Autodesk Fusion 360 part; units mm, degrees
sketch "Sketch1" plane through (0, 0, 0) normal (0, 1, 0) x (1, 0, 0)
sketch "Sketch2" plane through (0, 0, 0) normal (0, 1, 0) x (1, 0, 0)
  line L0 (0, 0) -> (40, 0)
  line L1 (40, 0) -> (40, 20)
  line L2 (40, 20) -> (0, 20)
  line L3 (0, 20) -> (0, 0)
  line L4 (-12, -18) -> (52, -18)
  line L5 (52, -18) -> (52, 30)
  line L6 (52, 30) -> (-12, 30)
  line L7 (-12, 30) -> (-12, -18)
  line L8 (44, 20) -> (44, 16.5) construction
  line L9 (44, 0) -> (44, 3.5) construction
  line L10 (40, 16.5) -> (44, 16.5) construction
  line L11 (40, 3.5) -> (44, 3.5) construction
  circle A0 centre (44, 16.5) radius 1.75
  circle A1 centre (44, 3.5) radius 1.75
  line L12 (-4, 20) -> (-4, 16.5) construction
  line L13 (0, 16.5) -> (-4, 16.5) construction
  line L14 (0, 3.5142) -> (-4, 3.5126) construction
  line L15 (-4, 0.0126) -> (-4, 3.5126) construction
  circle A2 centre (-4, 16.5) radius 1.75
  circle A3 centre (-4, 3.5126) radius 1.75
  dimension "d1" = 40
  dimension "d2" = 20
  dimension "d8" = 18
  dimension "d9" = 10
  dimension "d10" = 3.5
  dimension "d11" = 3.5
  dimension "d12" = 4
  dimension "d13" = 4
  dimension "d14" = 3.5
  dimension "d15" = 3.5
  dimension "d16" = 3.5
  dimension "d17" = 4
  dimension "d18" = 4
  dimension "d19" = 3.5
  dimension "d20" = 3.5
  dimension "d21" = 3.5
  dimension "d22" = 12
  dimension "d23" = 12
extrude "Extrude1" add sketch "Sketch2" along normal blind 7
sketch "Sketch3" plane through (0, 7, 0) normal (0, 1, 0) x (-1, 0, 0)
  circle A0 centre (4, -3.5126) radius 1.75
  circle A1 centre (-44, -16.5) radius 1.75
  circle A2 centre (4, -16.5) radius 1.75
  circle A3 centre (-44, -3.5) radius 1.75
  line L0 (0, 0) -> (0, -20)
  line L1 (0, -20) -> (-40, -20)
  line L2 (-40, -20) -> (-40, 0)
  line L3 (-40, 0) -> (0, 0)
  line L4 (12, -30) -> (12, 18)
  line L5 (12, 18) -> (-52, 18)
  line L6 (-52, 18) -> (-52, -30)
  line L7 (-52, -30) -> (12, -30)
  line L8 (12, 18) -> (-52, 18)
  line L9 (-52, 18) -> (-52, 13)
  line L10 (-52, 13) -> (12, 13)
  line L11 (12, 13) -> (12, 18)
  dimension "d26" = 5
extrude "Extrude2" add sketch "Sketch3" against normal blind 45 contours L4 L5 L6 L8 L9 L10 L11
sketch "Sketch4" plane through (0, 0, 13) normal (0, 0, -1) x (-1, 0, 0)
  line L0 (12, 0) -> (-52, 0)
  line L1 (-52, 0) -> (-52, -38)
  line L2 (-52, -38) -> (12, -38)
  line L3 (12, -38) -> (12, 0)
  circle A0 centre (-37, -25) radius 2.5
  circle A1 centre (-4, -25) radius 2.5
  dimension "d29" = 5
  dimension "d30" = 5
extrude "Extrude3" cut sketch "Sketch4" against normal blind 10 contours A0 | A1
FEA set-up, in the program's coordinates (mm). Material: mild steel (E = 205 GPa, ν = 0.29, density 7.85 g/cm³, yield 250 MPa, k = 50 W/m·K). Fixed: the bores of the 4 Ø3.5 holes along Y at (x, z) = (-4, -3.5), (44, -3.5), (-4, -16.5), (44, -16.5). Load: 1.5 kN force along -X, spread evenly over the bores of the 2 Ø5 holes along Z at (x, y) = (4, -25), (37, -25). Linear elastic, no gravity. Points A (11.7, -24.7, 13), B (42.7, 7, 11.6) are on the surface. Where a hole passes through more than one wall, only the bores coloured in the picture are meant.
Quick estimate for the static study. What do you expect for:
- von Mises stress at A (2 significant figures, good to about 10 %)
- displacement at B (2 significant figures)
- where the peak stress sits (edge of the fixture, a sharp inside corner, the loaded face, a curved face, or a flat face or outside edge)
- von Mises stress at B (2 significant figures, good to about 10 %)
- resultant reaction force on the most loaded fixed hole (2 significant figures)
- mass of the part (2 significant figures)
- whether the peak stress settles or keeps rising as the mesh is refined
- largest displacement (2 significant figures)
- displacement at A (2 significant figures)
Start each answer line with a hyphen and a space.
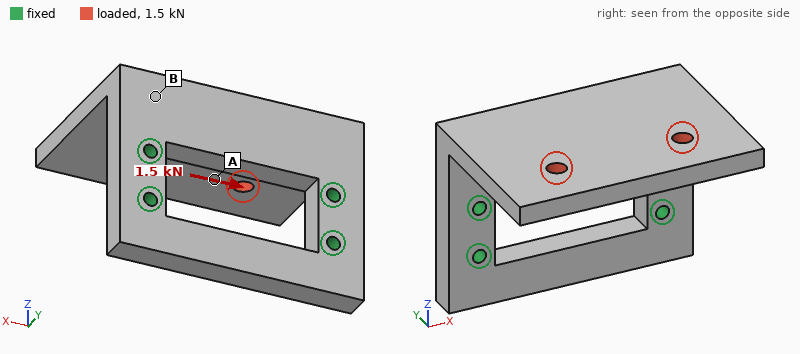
- 13 MPa
- 9.2 µm
- edge of the fixture
- 27 MPa
- 1.3 kN
- 220 g
- keeps rising
- 36 µm
- 20 µm
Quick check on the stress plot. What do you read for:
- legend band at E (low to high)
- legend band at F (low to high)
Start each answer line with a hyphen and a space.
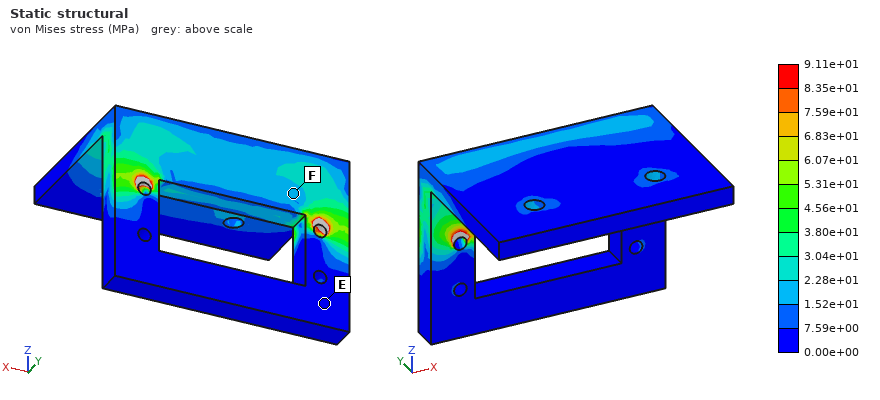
- 0.00e+00 to 7.59e+00 MPa
- 1.52e+01 to 2.28e+01 MPa
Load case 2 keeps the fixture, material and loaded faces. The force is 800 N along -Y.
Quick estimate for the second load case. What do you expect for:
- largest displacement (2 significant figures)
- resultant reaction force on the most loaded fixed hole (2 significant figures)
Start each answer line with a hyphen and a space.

- 40 µm
- 520 N
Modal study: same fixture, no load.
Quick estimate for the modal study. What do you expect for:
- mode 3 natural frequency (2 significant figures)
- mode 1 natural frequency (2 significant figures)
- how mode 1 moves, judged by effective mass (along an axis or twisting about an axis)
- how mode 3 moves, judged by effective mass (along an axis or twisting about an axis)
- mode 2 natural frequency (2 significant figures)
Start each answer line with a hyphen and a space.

- 5000 Hz
- 1600 Hz
- along Z
- along Y
- 3500 Hz
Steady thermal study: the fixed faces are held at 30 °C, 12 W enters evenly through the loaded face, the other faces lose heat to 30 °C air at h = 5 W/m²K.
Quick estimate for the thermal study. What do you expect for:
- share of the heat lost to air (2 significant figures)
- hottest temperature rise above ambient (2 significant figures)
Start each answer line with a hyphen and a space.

- 8.9 %
- 41 K
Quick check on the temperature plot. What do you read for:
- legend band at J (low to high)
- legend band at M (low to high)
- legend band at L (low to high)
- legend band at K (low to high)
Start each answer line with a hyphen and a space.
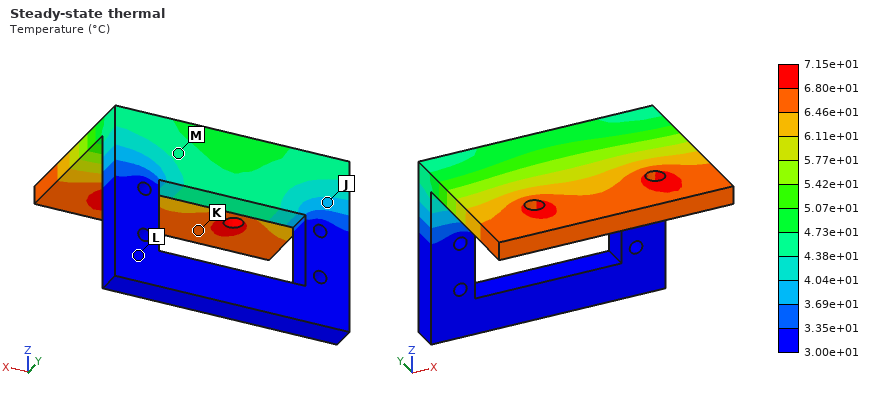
- 3.69e+01 to 4.04e+01 °C
- 4.38e+01 to 4.73e+01 °C
- 3.00e+01 to 3.35e+01 °C
- 6.46e+01 to 6.80e+01 °C
